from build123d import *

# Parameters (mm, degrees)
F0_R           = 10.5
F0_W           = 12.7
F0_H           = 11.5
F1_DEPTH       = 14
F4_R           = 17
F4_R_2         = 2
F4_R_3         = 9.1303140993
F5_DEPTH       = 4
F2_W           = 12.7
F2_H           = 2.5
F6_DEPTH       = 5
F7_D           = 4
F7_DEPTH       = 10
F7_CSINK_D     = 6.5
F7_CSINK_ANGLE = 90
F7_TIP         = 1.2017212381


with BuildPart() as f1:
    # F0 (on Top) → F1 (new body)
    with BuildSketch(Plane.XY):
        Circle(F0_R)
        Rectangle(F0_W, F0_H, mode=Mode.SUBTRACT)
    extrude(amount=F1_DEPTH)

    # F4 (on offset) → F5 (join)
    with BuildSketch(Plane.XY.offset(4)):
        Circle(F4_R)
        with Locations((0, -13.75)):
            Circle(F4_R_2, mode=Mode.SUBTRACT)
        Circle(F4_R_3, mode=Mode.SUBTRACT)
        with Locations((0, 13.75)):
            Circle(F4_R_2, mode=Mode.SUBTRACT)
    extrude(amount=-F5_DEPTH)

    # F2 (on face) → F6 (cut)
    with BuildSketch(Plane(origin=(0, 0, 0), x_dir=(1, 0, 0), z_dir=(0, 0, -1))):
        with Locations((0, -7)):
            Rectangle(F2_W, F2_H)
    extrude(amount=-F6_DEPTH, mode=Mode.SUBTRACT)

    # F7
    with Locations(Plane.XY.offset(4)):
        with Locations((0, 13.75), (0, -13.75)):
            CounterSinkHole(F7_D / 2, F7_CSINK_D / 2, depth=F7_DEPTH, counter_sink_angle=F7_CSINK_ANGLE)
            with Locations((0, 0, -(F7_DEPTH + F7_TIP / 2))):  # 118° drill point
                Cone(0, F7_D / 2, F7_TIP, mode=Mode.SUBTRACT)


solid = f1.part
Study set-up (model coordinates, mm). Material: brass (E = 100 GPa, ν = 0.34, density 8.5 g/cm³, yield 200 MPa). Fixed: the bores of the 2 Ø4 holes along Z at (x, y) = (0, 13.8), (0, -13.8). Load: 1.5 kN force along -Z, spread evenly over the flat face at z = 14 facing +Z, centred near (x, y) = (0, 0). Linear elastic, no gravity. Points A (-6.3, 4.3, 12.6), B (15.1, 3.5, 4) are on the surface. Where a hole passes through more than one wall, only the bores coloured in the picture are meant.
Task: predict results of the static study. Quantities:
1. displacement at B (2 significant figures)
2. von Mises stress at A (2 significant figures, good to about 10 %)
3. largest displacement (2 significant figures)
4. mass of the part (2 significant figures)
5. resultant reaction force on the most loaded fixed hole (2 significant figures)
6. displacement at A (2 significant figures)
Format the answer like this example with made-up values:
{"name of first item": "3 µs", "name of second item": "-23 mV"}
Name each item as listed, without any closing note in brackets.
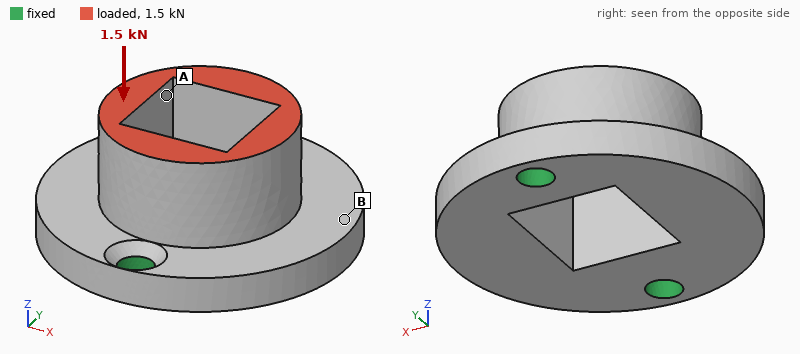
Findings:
{"displacement at B": "8.6 µm", "von Mises stress at A": "18 MPa", "largest displacement": "9.3 µm", "mass of the part": "41 g", "resultant reaction force on the most loaded fixed hole": "820 N", "displacement at A": "6.8 µm"}
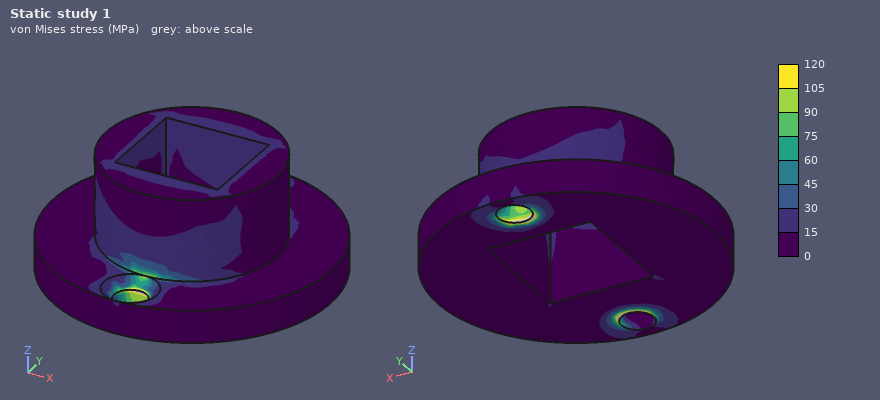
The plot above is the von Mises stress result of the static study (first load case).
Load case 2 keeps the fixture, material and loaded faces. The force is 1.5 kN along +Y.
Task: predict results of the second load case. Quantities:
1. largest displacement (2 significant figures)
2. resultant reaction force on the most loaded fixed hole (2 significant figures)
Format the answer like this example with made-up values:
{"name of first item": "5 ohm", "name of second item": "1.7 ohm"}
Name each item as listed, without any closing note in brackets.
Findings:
{"largest displacement": "15 µm", "resultant reaction force on the most loaded fixed hole": "1.1 kN"}
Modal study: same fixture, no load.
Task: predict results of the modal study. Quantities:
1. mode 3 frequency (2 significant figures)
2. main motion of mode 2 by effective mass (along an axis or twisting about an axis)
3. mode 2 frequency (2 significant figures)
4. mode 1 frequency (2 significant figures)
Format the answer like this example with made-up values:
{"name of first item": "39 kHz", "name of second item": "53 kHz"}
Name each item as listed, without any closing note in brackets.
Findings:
{"mode 3 frequency": "17 kHz", "main motion of mode 2 by effective mass": "along Z", "mode 2 frequency": "11 kHz", "mode 1 frequency": "5000 Hz"}
